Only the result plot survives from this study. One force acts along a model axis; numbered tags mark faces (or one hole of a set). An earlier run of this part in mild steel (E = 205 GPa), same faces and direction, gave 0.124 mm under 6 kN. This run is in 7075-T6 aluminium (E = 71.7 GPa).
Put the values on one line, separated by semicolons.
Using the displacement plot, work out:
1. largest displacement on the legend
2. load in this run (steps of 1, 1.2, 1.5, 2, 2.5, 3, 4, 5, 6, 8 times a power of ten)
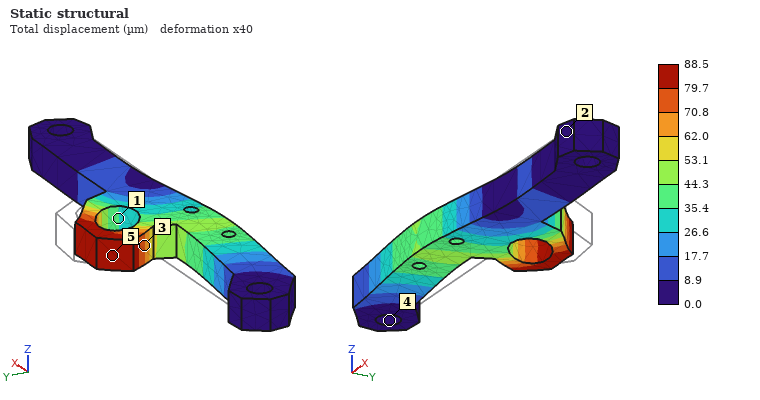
88.5 µm; 1.5 kN
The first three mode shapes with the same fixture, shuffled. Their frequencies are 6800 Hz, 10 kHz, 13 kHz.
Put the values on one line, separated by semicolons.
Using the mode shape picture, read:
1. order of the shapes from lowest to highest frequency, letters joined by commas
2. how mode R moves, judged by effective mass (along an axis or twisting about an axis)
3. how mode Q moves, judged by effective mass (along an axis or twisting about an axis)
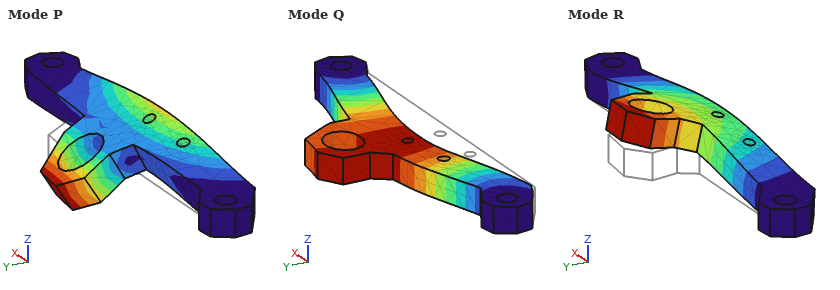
R, Q, P; along Z; along Y
